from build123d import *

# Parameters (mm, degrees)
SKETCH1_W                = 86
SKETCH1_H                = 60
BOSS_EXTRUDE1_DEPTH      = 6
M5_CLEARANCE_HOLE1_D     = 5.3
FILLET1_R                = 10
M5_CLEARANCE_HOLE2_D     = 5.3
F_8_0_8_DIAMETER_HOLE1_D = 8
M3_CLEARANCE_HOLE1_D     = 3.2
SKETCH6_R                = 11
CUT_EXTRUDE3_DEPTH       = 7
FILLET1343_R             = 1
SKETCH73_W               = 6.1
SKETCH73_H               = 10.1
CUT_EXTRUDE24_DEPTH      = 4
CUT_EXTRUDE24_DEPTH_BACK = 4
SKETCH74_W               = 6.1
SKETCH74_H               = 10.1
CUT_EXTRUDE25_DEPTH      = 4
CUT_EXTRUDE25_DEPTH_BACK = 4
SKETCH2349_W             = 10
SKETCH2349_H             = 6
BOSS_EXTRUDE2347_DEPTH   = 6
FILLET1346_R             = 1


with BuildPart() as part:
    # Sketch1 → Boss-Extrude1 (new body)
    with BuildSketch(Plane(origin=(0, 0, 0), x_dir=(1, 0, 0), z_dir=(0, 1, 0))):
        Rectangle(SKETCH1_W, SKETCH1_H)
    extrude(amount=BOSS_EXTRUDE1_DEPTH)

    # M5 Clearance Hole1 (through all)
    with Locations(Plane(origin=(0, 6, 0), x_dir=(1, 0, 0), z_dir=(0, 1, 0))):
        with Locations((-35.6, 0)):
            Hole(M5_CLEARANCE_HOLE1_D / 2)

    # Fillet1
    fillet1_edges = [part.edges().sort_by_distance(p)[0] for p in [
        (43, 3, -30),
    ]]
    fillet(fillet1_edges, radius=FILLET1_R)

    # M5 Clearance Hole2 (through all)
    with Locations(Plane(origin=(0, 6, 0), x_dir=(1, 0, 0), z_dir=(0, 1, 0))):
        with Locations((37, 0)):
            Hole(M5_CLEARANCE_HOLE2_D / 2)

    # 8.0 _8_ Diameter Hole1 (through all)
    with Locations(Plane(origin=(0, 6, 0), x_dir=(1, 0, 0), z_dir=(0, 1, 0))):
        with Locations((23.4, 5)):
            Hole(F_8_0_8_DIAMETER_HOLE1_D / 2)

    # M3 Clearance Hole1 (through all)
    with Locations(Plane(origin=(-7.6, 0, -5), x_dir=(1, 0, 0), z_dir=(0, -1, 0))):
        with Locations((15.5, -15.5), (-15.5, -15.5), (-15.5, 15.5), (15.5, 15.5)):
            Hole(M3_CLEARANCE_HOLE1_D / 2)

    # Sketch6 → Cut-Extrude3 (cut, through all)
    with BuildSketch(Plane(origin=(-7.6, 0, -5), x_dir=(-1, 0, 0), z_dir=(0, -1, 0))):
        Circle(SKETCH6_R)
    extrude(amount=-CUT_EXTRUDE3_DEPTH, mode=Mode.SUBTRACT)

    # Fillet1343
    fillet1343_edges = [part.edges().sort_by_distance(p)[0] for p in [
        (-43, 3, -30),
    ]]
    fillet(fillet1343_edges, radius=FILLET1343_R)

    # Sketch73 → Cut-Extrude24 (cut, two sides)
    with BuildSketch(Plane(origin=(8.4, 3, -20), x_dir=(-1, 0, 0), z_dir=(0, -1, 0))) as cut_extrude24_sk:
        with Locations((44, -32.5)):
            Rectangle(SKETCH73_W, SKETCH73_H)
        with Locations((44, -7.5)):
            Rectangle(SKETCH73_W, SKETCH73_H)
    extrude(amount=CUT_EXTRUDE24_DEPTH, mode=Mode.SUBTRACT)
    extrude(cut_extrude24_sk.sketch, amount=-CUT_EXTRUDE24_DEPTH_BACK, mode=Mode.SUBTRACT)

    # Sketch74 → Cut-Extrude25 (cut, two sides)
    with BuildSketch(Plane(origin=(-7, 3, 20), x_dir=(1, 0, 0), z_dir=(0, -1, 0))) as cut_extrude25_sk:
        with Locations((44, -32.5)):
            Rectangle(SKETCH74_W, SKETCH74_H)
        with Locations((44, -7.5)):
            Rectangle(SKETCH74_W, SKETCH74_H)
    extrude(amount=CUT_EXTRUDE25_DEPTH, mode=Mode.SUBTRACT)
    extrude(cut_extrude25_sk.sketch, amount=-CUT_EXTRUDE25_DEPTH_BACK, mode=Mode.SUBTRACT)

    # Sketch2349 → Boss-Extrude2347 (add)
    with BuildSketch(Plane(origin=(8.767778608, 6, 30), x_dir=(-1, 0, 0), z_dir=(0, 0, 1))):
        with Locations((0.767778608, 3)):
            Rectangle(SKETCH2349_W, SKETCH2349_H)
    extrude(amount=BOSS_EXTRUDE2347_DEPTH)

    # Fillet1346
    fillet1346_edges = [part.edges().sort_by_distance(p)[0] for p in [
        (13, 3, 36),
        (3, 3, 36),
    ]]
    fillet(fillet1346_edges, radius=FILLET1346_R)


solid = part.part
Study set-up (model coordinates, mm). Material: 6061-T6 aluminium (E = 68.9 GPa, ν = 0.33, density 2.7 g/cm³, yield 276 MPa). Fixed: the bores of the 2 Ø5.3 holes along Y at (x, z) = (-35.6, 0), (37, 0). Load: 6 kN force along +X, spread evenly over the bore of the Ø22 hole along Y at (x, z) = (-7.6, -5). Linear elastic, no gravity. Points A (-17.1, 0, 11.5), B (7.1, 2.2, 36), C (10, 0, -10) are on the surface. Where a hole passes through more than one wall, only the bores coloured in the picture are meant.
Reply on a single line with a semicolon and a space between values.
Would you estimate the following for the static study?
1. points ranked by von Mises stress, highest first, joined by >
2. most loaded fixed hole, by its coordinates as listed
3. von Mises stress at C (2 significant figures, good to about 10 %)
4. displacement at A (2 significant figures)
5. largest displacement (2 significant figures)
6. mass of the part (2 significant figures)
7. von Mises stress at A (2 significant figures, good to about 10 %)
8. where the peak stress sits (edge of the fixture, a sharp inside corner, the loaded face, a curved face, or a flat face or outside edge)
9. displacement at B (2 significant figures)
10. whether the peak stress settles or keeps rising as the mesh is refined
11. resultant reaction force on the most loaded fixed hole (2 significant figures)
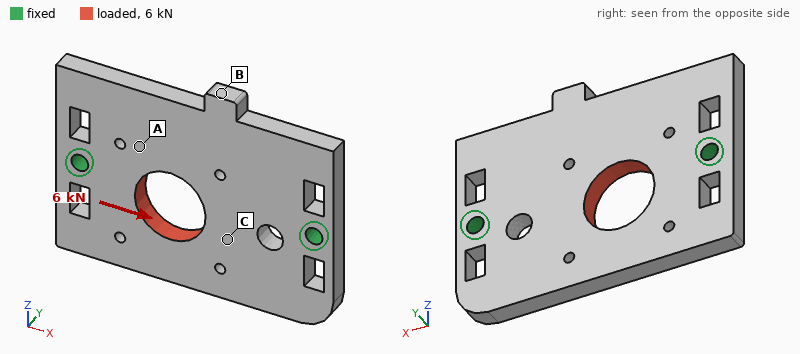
C > A > B; (-35.6, 0); 17 MPa; 7.6 µm; 18 µm; 72 g; 10 MPa; edge of the fixture; 5.2 µm; keeps rising; 3.3 kN
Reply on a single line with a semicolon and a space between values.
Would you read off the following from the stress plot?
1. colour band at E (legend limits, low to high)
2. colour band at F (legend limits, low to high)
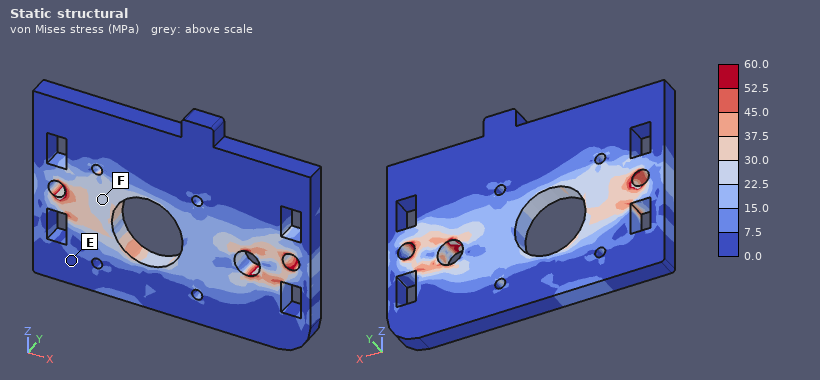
0.0 to 7.5 MPa; 22.5 to 30.0 MPa
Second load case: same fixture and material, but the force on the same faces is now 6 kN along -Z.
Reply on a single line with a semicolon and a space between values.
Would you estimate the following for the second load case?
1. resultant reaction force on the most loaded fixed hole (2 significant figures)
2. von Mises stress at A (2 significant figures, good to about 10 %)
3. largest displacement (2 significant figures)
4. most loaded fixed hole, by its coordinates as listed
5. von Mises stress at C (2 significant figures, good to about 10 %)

3.7 kN; 22 MPa; 24 µm; (-35.6, 0); 16 MPa
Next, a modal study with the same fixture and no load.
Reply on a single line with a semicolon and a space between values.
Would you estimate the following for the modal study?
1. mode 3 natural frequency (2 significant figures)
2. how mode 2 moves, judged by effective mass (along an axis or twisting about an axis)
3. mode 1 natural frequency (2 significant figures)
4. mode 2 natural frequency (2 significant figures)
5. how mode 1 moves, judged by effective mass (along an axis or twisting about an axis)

5700 Hz; along Y; 2600 Hz; 3400 Hz; twisting about X
